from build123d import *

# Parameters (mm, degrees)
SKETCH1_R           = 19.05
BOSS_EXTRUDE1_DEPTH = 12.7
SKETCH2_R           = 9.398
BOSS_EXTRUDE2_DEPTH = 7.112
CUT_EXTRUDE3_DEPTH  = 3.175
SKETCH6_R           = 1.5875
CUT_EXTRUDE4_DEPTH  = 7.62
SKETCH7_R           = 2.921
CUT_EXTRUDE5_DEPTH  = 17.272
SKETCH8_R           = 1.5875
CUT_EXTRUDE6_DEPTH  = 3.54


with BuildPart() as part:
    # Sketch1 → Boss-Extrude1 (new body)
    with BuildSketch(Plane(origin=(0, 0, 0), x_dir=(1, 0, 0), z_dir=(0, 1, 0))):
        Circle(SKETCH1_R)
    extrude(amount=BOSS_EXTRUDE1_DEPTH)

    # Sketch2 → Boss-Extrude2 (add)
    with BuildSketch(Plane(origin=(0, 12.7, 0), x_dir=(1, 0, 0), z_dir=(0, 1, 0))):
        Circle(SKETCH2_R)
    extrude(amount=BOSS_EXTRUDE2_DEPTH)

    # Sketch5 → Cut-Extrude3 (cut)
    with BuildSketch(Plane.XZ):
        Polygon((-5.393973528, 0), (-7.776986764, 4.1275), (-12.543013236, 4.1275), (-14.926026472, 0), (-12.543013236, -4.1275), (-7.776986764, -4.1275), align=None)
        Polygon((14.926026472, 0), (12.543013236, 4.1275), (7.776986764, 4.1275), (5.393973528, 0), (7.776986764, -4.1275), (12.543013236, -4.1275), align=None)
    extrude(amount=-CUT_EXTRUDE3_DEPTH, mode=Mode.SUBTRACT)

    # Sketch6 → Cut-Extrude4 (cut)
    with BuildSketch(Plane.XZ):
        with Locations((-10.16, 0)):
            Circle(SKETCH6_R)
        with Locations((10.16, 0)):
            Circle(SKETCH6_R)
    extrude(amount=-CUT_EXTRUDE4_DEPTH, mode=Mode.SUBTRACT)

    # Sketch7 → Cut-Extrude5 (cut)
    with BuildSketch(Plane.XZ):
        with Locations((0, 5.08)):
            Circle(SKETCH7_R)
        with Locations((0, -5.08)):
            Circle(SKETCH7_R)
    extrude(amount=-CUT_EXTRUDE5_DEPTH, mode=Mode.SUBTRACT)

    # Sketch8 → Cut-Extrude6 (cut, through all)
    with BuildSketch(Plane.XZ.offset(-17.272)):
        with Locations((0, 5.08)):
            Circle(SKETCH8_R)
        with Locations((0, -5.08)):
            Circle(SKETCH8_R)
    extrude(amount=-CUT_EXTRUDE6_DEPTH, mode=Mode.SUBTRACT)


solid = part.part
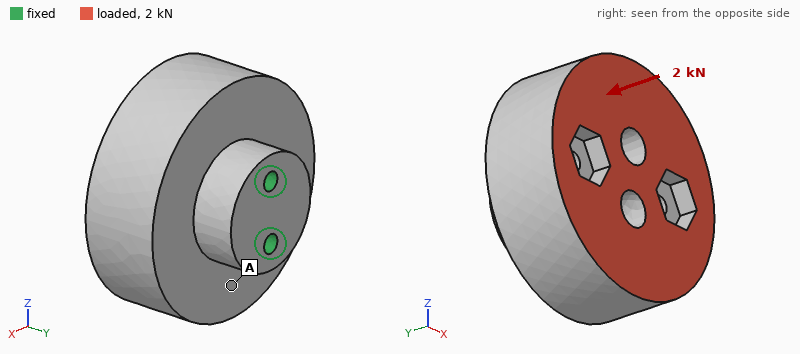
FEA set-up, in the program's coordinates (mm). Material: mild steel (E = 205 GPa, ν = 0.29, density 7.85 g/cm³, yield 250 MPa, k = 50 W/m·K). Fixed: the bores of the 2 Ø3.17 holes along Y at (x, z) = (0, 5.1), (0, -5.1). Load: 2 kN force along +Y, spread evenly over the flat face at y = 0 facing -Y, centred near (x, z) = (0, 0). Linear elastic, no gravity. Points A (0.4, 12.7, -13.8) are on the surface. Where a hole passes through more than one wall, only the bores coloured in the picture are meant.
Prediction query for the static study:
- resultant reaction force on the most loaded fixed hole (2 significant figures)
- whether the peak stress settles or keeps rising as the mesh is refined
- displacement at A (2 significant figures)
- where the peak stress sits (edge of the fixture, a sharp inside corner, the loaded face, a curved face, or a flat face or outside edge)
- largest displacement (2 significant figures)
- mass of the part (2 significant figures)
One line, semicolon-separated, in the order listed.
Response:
1.0 kN; keeps rising; 1.8 µm; edge of the fixture; 2.1 µm; 120 g
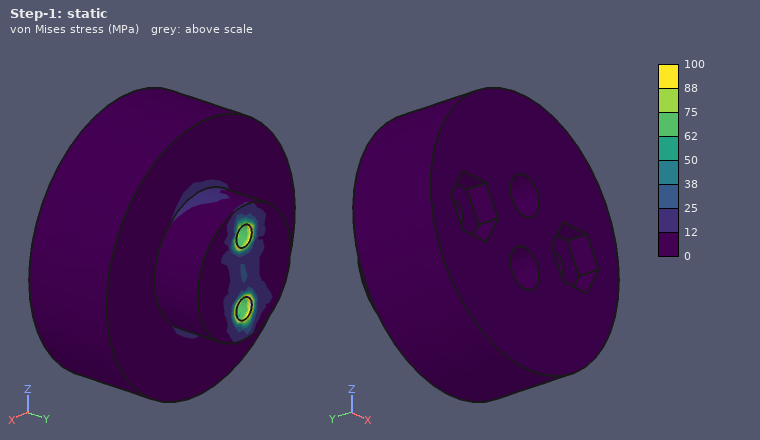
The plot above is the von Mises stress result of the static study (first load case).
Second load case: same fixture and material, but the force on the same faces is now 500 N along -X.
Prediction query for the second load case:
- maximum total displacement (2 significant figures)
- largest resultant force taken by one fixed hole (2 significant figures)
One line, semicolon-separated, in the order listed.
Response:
30 µm; 250 N
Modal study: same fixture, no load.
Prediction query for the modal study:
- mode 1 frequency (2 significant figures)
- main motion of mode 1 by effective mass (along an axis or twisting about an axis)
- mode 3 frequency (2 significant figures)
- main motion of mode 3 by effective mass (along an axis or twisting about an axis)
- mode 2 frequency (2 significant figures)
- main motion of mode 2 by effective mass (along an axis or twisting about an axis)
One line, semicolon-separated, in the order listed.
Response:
2800 Hz; along X; 7800 Hz; twisting about Y; 6100 Hz; along Z
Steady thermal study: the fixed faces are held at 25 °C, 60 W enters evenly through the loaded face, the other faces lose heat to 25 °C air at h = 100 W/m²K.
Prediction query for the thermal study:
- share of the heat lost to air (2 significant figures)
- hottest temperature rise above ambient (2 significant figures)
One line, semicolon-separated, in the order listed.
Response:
36 %; 68 K
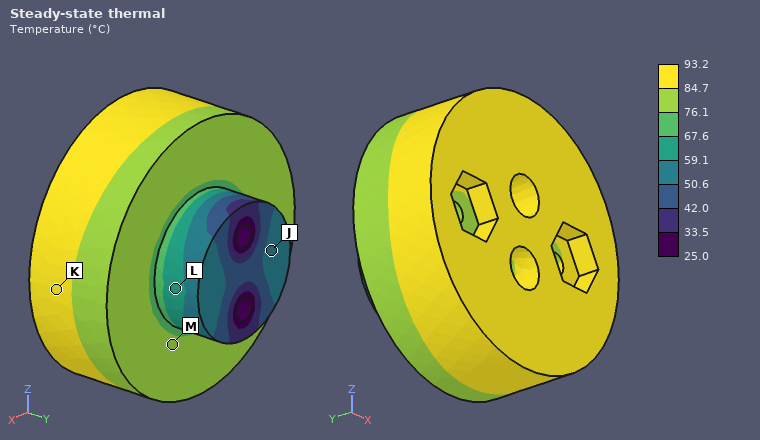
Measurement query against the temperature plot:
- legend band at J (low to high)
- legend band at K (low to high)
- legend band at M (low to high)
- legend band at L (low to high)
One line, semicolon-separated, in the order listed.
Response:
50.6 to 59.1 °C; 84.7 to 93.2 °C; 76.1 to 84.7 °C; 59.1 to 67.6 °C
